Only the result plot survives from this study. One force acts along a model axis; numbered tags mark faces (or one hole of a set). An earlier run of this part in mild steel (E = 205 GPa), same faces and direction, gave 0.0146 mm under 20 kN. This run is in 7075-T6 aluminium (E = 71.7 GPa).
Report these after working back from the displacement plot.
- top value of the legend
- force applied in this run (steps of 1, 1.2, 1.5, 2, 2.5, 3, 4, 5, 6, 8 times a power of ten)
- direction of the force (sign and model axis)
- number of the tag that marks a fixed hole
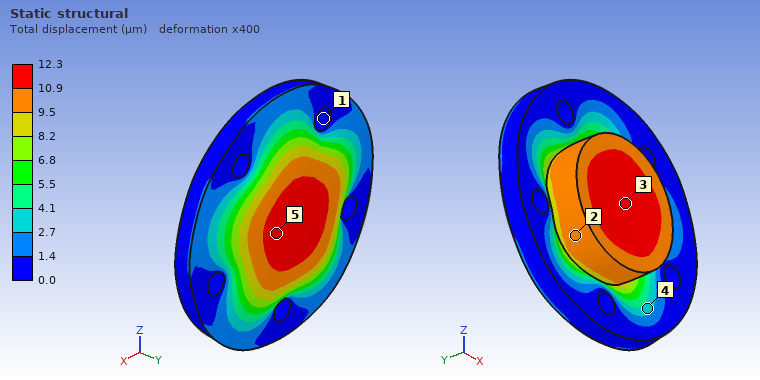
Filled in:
12.3 µm
6 kN
+Y
1
